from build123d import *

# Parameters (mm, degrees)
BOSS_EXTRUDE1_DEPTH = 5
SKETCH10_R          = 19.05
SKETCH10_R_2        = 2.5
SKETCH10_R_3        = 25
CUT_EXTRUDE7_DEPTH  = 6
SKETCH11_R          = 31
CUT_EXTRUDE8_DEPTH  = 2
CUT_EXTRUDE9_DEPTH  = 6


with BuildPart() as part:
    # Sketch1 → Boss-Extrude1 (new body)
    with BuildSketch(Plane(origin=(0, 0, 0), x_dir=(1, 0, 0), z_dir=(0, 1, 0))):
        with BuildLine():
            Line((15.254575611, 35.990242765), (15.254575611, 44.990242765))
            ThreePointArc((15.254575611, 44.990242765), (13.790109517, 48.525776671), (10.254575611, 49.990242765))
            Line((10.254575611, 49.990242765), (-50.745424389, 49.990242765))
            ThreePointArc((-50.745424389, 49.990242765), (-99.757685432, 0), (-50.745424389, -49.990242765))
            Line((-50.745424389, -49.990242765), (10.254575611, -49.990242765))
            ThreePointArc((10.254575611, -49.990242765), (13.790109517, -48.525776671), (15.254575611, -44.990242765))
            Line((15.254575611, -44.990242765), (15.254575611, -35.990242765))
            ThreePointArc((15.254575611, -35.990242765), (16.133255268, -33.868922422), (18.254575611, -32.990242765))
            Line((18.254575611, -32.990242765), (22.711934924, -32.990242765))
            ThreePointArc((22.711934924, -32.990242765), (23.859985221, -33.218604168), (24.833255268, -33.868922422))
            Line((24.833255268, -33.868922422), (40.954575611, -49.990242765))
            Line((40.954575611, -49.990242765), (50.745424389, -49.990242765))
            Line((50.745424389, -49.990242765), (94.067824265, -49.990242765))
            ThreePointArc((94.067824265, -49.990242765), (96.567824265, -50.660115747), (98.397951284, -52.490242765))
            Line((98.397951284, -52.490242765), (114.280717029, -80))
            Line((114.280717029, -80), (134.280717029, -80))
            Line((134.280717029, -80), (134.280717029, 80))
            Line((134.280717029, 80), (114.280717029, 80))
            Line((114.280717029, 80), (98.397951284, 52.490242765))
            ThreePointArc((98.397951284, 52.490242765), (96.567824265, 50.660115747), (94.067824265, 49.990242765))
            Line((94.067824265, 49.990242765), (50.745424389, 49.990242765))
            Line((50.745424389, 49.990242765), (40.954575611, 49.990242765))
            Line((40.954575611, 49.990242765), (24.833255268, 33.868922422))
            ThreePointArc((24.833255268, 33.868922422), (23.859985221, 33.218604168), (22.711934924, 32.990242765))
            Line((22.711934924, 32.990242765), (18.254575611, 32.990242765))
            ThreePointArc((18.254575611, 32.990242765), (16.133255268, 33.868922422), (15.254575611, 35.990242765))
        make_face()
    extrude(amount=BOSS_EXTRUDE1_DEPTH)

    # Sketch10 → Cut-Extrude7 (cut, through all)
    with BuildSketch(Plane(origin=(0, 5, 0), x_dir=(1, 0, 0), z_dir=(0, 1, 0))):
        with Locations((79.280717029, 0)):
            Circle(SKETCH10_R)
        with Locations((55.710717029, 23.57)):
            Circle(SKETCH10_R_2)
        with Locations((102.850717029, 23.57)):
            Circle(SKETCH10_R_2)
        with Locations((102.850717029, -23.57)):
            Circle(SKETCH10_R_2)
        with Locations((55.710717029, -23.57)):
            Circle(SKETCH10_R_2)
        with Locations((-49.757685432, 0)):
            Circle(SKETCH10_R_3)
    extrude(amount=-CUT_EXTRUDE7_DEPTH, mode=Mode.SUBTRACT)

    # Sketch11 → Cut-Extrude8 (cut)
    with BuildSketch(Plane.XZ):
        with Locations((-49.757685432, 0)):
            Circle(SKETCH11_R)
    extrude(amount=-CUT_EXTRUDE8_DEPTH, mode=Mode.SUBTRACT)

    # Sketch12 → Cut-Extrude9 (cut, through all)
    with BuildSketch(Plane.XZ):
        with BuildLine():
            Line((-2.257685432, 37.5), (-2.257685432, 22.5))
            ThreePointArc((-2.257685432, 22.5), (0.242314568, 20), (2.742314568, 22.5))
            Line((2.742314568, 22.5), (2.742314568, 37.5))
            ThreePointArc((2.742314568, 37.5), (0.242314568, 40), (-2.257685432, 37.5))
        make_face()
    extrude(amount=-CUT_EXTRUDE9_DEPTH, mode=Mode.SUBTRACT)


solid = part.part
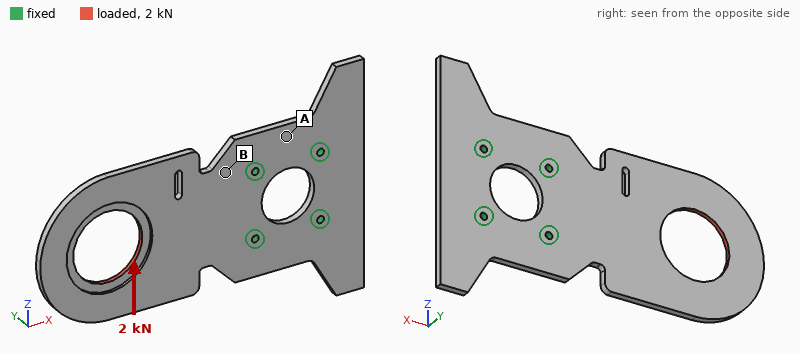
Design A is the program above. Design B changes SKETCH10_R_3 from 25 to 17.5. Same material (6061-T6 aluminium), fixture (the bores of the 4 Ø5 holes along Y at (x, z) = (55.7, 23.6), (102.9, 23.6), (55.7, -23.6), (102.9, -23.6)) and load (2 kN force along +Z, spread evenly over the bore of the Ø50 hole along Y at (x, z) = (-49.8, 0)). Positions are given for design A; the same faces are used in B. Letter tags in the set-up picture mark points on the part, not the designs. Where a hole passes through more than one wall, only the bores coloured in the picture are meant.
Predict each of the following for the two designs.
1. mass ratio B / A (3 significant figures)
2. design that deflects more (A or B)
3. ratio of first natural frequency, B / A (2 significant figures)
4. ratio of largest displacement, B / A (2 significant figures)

1.03
A
0.96
0.90
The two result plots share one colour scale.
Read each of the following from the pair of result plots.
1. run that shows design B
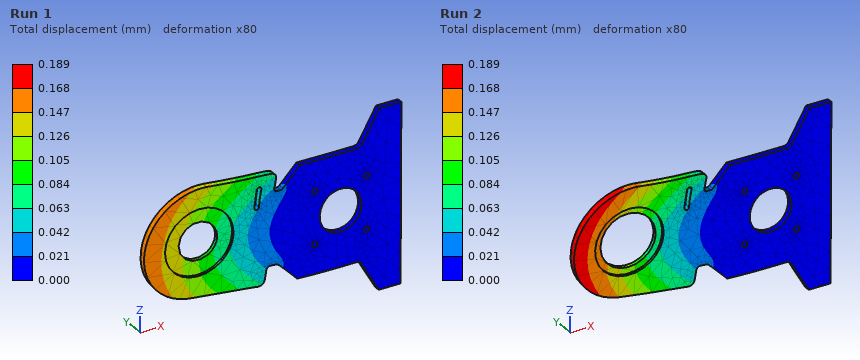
Run 1
